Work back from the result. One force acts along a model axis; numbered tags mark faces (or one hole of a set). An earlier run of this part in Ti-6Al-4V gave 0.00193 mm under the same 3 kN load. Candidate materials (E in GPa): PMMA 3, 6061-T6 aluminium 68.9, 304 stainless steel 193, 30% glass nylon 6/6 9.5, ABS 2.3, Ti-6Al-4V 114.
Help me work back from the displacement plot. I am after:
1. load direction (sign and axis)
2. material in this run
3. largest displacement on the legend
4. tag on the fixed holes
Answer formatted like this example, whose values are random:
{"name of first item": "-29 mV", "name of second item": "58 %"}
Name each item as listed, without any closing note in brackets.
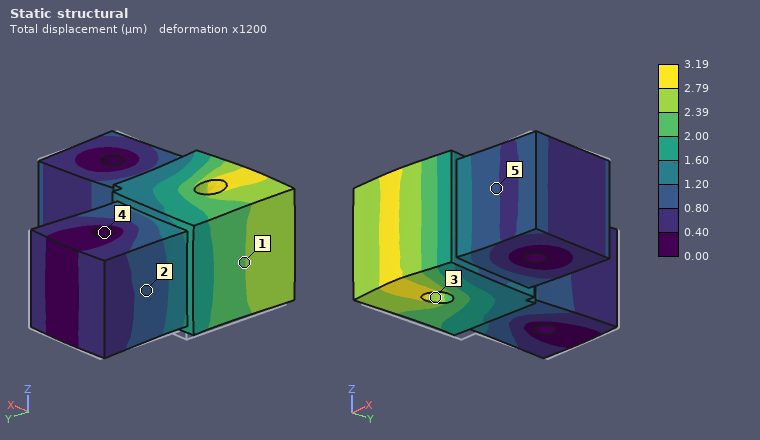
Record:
{"load direction": "-Y", "material in this run": "6061-T6 aluminium", "largest displacement on the legend": "3.19 µm", "tag on the fixed holes": "4"}
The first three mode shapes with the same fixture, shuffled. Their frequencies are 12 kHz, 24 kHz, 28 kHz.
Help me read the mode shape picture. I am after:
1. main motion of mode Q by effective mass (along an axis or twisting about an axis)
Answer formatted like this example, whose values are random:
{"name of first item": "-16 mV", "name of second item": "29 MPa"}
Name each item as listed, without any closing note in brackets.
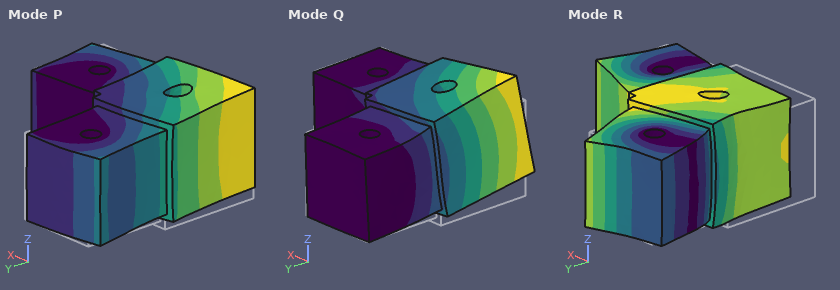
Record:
{"main motion of mode Q by effective mass": "along Z"}
